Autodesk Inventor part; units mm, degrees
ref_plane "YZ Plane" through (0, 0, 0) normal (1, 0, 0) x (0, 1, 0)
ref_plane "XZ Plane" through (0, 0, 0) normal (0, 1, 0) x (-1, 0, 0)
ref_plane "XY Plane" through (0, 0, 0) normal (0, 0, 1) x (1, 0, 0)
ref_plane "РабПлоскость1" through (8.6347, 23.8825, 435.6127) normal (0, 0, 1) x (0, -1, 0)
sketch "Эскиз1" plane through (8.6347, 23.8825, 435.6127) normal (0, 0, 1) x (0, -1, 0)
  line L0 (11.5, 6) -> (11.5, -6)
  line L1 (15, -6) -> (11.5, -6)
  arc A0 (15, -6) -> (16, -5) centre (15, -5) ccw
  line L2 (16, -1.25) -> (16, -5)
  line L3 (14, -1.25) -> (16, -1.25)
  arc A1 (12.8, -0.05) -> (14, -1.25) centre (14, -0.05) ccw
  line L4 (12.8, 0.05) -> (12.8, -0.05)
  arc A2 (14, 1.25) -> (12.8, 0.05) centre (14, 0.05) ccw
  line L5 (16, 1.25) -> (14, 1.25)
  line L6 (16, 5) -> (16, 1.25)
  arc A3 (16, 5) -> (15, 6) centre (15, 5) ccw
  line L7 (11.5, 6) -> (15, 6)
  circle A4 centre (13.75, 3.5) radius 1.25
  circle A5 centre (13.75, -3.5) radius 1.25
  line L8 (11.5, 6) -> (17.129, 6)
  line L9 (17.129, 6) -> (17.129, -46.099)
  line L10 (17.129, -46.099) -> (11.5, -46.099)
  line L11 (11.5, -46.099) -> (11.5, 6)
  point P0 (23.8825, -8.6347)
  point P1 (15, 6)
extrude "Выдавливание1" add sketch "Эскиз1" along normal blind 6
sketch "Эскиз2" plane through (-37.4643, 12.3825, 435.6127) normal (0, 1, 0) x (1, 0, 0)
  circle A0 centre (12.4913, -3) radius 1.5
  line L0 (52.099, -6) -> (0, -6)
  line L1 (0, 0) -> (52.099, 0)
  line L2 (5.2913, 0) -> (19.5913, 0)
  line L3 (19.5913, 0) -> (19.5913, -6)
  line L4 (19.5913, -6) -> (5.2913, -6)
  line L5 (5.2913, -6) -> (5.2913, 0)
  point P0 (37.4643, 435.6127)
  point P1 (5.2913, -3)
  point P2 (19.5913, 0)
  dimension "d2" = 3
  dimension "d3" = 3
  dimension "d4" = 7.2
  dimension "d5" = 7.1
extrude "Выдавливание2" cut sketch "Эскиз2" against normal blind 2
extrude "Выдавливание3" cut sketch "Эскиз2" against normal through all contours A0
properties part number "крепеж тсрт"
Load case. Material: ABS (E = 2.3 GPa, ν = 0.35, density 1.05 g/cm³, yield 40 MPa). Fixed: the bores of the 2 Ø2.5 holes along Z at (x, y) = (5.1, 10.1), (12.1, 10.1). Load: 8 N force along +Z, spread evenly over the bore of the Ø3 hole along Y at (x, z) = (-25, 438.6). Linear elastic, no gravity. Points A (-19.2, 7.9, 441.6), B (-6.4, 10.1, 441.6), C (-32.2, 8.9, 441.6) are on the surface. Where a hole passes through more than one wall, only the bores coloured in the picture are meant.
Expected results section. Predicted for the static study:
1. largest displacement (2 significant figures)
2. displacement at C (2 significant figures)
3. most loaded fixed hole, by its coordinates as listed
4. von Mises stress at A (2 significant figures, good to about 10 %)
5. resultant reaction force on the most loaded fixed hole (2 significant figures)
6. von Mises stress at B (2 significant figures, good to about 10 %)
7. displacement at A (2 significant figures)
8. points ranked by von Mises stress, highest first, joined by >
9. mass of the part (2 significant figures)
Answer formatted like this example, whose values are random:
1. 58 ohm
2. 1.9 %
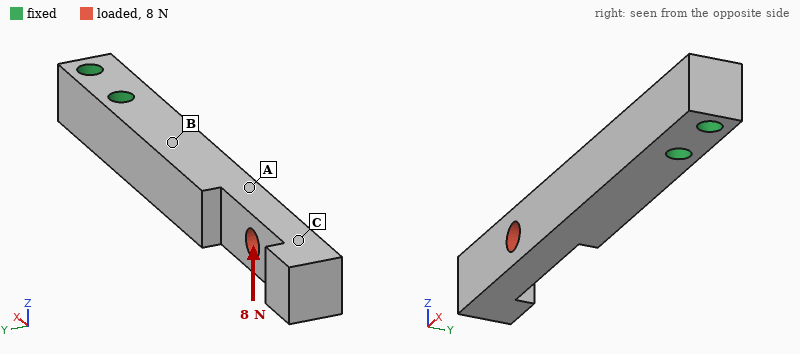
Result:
1. 0.52 mm
2. 0.43 mm
3. (5.1, 10.1)
4. 2.0 MPa
5. 10 N
6. 4.4 MPa
7. 0.23 mm
8. B > A > C
9. 1.6 g
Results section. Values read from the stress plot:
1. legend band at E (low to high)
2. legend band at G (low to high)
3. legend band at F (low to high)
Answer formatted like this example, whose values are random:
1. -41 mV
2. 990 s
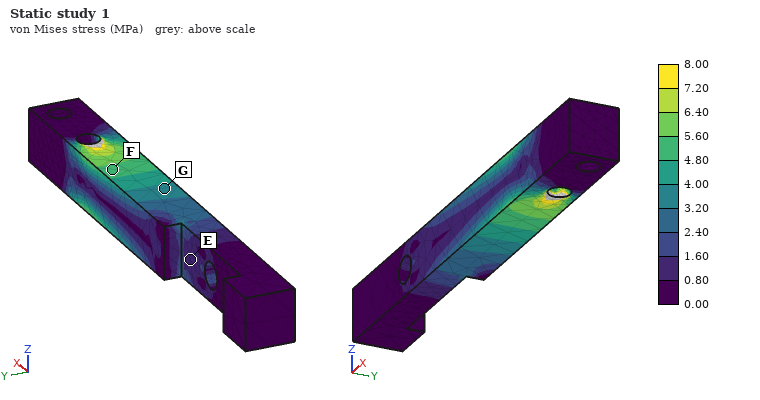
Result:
1. 0.80 to 1.60 MPa
2. 3.20 to 4.00 MPa
3. 4.80 to 5.60 MPa
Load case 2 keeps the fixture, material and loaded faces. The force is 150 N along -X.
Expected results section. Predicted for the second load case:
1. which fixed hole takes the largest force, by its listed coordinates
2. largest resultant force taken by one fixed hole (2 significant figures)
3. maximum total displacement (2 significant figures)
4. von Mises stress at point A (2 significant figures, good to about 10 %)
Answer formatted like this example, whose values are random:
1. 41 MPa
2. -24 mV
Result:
1. (5.1, 10.1)
2. 130 N
3. 0.58 mm
4. 7.1 MPa
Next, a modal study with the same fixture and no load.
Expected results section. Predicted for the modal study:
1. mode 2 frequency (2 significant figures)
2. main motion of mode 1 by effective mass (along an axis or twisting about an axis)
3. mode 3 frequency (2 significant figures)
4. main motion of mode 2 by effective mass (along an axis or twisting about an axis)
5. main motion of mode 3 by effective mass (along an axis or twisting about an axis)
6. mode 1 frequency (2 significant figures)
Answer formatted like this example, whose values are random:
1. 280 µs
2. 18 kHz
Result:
1. 870 Hz
2. along Y
3. 3000 Hz
4. along Z
5. along Y
6. 740 Hz
